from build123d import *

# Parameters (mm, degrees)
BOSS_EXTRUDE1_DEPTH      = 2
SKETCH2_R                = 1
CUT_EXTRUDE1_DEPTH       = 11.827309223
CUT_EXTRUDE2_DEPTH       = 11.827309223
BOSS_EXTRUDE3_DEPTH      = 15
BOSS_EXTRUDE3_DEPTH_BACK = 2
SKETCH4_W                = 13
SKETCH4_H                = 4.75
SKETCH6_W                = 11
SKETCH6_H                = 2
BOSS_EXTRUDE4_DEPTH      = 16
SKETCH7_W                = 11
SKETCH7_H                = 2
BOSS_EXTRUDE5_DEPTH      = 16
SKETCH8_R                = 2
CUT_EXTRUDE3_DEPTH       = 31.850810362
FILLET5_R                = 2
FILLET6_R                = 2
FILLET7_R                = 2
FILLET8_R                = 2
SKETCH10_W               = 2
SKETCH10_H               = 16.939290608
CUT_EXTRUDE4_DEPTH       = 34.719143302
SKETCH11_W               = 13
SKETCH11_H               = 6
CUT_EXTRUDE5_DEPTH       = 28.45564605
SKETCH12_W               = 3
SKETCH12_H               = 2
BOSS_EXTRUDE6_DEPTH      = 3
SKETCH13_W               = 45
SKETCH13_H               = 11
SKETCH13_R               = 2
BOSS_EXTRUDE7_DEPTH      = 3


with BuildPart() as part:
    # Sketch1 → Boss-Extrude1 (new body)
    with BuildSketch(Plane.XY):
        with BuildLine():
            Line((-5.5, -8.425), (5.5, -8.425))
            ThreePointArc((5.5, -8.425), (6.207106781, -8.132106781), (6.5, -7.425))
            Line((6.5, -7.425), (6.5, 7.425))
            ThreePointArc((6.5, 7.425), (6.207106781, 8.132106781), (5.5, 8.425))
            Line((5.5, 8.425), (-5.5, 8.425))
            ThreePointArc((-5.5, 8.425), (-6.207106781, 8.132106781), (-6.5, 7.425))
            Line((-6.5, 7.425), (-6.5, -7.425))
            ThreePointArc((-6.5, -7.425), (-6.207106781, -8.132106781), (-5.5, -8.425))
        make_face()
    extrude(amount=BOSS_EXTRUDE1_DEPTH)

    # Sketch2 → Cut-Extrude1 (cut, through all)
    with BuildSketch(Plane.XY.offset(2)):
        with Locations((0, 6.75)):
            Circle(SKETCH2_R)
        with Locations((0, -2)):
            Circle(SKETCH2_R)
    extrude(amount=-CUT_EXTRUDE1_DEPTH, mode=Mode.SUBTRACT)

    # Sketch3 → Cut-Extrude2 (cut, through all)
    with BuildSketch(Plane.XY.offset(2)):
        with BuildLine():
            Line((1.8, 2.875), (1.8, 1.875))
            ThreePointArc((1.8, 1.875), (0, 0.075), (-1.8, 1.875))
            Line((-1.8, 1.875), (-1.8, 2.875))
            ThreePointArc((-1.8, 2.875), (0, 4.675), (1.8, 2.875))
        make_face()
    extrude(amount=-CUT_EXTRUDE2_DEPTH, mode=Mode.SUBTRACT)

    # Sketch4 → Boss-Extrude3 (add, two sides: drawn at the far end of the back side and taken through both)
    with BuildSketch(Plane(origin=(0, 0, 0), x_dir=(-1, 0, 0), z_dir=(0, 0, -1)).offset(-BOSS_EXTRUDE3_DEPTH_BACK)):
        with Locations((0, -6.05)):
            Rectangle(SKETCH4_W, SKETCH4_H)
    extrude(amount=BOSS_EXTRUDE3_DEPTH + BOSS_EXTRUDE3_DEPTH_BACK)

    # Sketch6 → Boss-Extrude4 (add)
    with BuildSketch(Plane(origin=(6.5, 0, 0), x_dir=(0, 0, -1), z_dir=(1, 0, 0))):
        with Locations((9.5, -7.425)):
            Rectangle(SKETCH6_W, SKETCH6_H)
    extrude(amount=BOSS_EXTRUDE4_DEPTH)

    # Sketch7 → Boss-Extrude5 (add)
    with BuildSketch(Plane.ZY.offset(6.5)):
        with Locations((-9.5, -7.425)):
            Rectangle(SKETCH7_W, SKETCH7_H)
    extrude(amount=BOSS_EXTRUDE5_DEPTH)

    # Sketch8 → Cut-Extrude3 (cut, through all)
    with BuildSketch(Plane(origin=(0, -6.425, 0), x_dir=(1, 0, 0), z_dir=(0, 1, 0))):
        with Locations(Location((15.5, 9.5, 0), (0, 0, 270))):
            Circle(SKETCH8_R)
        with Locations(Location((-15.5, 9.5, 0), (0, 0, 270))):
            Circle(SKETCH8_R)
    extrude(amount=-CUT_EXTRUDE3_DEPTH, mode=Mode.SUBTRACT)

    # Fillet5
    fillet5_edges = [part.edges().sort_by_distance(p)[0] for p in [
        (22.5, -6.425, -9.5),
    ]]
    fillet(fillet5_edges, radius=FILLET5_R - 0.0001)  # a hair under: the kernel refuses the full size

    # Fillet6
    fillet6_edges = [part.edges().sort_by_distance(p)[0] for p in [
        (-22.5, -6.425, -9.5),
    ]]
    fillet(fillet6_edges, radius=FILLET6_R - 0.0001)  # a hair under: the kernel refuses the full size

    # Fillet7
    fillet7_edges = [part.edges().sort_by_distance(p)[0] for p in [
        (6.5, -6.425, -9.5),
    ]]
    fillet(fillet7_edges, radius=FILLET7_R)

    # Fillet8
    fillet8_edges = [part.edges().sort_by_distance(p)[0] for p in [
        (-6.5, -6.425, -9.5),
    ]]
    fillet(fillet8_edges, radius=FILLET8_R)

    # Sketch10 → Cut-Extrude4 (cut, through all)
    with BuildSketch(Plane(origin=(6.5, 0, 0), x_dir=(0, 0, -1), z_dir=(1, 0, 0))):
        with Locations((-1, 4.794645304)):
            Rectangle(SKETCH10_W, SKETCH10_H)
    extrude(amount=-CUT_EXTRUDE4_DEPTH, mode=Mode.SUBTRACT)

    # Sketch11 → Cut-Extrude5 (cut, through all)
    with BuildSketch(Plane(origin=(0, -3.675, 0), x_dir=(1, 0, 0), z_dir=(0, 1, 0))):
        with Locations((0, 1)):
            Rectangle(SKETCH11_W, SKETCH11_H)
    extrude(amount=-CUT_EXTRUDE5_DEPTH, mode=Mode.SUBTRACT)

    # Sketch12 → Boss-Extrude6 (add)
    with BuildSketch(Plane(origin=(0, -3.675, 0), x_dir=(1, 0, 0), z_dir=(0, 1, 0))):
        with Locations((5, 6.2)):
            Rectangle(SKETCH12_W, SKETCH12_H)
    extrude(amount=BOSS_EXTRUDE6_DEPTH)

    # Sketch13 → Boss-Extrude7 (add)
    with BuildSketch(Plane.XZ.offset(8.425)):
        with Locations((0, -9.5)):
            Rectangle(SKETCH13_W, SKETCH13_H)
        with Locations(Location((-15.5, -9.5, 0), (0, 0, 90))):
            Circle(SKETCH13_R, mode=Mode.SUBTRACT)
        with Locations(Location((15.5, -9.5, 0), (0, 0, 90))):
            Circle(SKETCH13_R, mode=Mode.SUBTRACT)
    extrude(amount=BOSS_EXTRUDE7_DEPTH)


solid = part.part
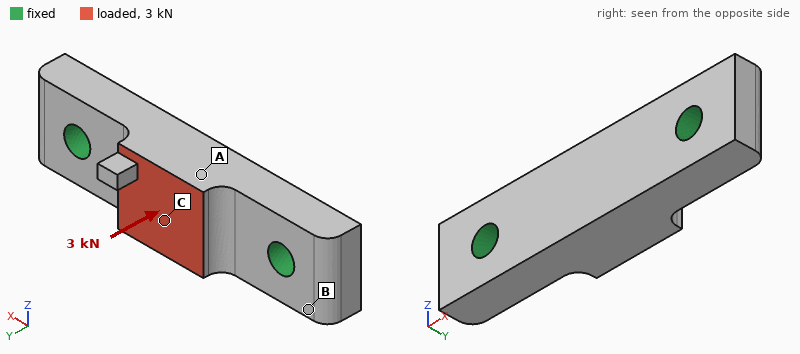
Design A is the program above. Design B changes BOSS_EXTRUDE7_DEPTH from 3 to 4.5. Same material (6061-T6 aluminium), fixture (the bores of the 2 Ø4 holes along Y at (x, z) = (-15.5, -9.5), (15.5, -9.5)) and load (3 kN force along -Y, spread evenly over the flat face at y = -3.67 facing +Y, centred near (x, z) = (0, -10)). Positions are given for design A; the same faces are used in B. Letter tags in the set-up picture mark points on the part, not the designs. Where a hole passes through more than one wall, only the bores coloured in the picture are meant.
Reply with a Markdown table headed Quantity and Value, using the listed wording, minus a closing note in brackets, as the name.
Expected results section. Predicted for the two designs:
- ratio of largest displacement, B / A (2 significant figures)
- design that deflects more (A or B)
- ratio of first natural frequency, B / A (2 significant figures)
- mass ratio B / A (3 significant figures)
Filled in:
| Quantity | Value |
|---|---|
| ratio of largest displacement, B / A | 0.64 |
| design that deflects more | A |
| ratio of first natural frequency, B / A | 1.1 |
| mass ratio B / A | 1.26 |
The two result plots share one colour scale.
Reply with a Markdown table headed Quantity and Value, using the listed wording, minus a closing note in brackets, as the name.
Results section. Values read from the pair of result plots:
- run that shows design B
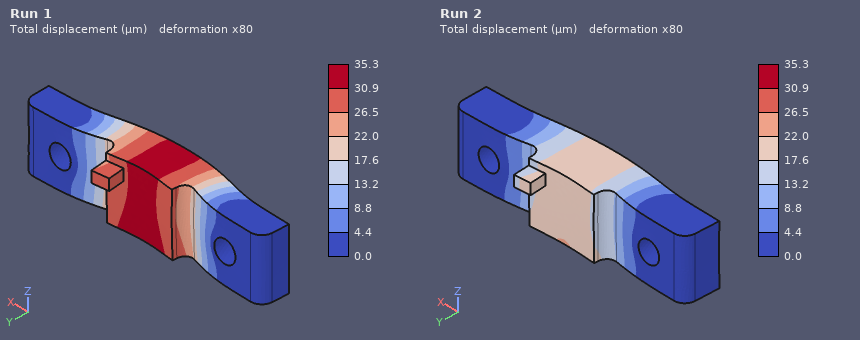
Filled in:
| Quantity | Value |
|---|---|
| run that shows design B | Run 2 |
